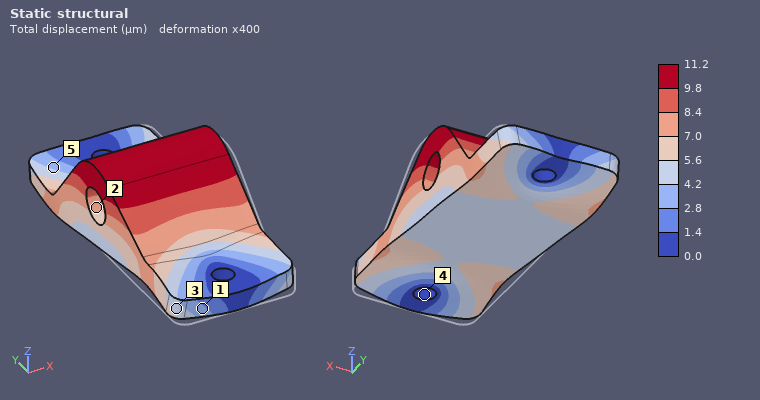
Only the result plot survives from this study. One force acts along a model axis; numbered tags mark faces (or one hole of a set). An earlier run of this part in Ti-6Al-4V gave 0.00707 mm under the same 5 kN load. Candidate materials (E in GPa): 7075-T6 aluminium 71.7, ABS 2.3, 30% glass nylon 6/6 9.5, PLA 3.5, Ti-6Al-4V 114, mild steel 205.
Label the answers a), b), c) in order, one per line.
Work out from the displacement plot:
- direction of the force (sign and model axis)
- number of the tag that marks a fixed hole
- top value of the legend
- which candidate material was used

a) +Y
b) 4
c) 11.2 µm
d) 7075-T6 aluminium
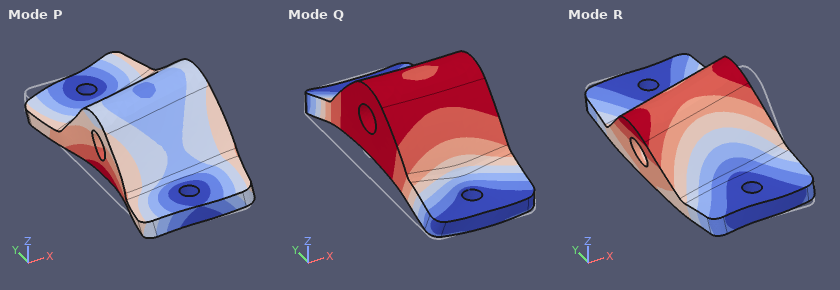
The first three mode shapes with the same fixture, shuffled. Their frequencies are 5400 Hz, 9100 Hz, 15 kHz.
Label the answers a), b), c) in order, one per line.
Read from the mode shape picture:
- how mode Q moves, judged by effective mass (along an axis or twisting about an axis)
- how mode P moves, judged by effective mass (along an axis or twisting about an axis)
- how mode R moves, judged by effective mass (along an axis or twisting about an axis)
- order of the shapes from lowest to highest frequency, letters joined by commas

a) along Z
b) along X
c) along X
d) R, Q, P
